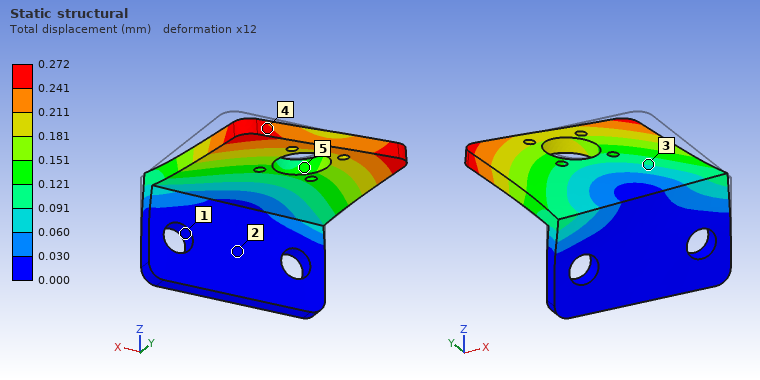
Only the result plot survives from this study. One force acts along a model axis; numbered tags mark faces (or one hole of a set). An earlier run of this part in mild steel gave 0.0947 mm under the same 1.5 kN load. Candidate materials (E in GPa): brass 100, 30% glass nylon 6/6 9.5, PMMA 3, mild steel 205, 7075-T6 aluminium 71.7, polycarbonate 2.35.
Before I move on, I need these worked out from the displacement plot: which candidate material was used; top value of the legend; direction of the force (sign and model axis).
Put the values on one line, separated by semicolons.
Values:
7075-T6 aluminium; 0.272 mm; -X
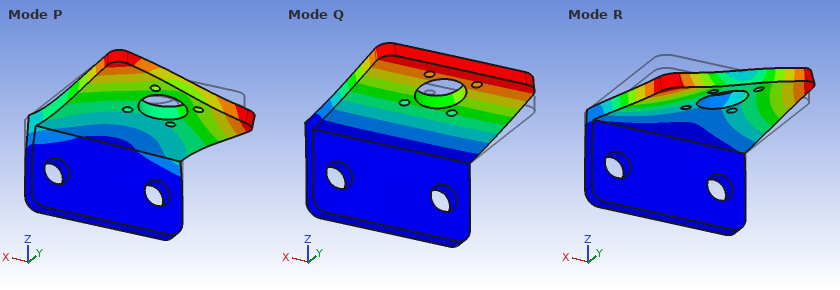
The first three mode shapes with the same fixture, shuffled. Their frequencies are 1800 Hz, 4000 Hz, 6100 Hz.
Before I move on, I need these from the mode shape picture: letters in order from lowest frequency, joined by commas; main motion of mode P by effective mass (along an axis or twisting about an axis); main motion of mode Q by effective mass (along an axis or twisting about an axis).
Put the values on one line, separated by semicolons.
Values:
Q, R, P; along X; along Z
